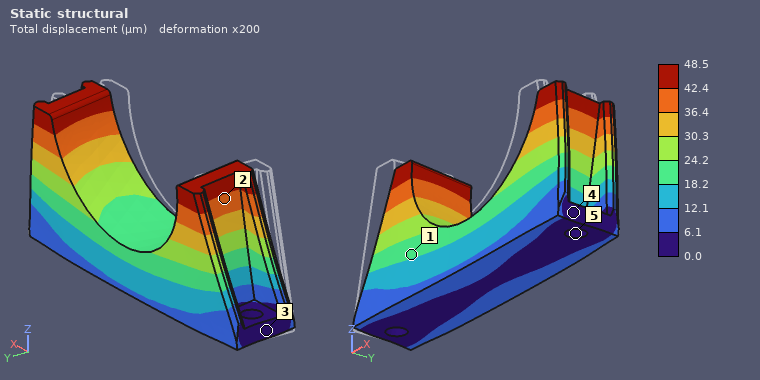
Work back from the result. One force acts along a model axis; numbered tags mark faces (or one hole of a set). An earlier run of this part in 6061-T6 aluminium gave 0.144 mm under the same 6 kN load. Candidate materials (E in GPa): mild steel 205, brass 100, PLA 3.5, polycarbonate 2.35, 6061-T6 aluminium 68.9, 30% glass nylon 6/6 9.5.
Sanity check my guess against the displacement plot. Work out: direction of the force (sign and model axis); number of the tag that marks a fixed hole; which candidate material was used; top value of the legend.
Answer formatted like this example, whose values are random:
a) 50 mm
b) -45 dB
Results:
a) +Y
b) 5
c) mild steel
d) 48.5 µm
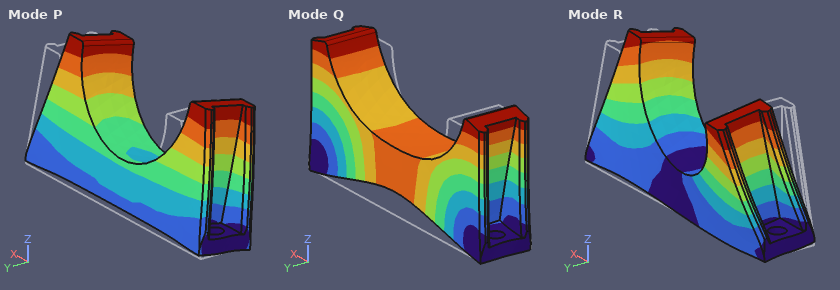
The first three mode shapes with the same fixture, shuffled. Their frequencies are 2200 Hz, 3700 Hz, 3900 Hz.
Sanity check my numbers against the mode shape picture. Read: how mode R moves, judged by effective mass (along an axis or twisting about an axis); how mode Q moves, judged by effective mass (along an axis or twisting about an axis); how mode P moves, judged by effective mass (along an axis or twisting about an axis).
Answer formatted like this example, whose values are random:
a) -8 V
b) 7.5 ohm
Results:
a) twisting about Z
b) along Z
c) along Y
